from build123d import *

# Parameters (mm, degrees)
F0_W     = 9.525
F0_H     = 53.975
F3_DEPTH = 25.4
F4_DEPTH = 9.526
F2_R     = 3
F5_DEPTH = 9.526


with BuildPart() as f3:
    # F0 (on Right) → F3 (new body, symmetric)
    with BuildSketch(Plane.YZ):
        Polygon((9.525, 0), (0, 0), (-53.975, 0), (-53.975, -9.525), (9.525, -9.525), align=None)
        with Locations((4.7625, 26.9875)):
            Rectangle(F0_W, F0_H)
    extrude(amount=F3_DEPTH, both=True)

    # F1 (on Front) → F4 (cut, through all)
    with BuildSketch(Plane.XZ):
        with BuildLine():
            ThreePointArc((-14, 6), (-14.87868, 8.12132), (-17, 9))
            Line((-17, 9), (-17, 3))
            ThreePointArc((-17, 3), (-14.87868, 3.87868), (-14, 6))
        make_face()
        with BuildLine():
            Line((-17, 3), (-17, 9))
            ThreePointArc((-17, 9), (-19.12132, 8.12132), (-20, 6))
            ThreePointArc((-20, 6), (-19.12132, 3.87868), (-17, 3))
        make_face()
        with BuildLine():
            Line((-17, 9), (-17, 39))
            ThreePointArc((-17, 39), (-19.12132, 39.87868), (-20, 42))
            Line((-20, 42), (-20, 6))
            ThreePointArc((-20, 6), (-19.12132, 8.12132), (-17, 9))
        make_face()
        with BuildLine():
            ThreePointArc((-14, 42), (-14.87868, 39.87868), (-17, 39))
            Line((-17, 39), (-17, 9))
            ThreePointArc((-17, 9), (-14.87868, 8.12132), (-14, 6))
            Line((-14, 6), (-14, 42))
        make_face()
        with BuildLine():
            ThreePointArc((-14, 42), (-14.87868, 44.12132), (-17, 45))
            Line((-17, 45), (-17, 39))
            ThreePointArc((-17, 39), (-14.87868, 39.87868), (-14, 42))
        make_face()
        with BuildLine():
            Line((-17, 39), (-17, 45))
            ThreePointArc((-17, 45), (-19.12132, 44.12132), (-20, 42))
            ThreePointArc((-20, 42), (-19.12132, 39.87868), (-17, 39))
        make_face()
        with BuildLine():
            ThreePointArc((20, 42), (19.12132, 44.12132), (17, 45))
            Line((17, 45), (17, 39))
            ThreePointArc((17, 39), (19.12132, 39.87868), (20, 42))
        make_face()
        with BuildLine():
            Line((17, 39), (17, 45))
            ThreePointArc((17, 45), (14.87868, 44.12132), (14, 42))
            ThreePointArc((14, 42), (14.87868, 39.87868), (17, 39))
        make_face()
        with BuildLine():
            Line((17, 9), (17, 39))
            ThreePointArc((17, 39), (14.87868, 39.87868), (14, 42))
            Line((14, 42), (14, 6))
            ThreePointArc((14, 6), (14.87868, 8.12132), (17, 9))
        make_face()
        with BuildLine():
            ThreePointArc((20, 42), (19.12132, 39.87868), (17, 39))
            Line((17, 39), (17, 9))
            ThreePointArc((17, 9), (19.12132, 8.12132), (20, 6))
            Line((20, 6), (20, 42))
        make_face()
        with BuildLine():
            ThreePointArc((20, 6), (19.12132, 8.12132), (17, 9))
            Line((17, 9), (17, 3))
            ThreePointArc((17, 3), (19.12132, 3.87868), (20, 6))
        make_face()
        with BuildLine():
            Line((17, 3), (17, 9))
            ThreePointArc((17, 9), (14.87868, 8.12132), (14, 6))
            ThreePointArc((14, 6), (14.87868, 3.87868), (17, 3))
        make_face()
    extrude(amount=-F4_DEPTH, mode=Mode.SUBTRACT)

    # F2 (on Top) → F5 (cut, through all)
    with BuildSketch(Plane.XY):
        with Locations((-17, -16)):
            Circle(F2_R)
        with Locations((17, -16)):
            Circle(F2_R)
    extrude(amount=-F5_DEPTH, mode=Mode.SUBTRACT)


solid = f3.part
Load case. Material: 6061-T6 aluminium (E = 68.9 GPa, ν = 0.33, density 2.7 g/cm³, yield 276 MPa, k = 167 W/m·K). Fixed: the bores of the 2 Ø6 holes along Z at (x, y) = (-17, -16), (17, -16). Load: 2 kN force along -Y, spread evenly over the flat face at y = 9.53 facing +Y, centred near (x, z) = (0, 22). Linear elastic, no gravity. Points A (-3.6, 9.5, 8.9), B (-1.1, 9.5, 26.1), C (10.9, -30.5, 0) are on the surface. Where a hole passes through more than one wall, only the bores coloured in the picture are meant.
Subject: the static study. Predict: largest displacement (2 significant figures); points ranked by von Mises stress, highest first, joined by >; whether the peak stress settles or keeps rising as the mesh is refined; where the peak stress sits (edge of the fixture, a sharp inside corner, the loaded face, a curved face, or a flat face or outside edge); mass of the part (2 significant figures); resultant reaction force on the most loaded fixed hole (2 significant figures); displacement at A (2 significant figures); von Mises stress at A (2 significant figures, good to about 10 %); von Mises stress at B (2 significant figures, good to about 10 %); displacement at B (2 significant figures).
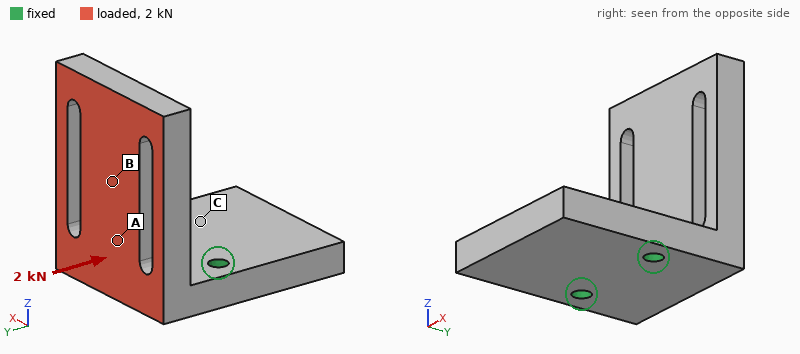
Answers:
0.45 mm
A > B > C
keeps rising
edge of the fixture
140 g
1.0 kN
0.11 mm
47 MPa
22 MPa
0.22 mm
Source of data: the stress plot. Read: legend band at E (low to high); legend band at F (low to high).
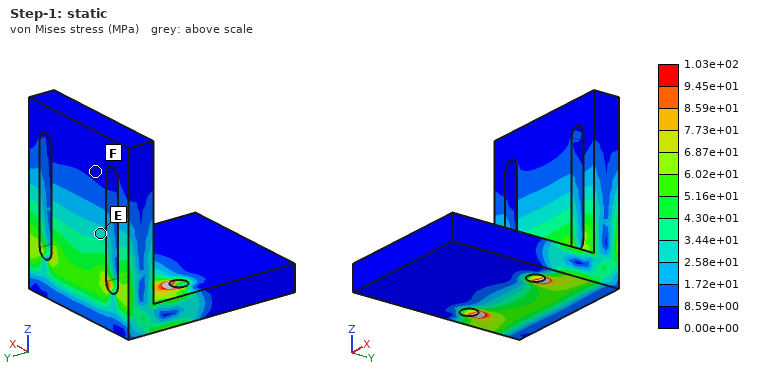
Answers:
2.58e+01 to 3.44e+01 MPa
0.00e+00 to 8.59e+00 MPa
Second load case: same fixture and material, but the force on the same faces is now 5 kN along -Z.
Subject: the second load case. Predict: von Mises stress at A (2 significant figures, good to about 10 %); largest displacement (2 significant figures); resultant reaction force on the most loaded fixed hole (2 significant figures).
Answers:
31 MPa
0.51 mm
2.5 kN
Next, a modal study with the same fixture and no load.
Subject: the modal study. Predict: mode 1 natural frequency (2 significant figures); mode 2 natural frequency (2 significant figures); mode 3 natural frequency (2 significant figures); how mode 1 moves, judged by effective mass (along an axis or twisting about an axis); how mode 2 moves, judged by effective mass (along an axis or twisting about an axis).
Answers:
1500 Hz
3100 Hz
4900 Hz
along Y
along X
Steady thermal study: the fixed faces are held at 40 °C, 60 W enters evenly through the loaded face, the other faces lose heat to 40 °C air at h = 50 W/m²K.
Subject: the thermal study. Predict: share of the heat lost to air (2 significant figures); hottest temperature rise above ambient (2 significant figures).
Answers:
14 %
33 K
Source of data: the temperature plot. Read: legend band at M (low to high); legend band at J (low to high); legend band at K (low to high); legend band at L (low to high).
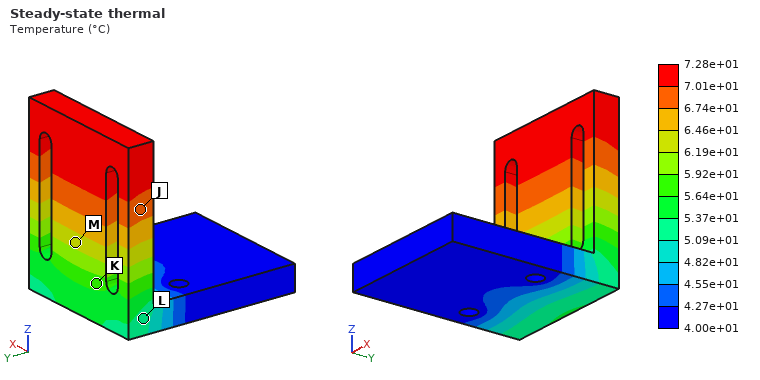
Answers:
6.19e+01 to 6.46e+01 °C
6.74e+01 to 7.01e+01 °C
5.64e+01 to 5.92e+01 °C
5.09e+01 to 5.37e+01 °C
